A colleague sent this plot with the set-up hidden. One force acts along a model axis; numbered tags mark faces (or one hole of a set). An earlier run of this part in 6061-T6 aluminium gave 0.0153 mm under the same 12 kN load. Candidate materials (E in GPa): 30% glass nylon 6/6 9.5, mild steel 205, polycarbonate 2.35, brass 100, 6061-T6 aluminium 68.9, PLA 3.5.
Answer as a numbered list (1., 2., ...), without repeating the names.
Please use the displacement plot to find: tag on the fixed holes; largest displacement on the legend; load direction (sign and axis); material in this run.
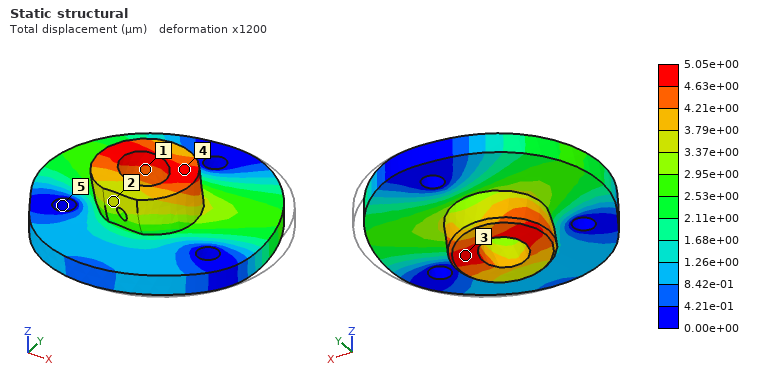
1. 5
2. 5.05e+00 µm
3. -X
4. mild steel
